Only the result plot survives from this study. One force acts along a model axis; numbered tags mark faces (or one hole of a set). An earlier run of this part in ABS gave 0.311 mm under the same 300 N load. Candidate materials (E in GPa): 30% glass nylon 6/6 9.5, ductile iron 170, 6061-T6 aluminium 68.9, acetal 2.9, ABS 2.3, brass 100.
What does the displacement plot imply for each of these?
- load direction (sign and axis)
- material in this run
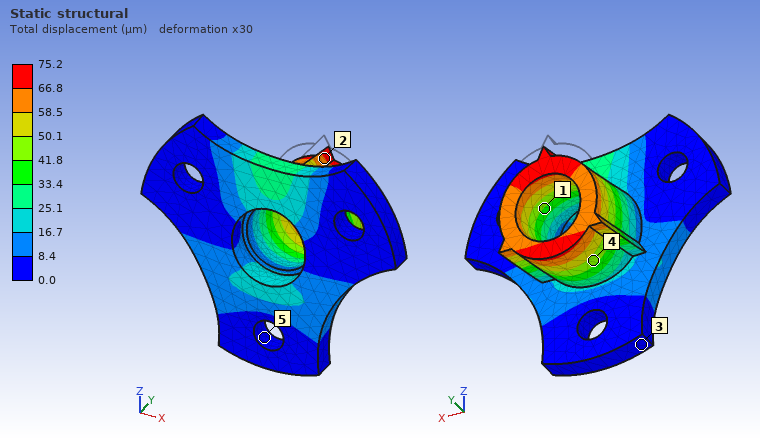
-Z
30% glass nylon 6/6
